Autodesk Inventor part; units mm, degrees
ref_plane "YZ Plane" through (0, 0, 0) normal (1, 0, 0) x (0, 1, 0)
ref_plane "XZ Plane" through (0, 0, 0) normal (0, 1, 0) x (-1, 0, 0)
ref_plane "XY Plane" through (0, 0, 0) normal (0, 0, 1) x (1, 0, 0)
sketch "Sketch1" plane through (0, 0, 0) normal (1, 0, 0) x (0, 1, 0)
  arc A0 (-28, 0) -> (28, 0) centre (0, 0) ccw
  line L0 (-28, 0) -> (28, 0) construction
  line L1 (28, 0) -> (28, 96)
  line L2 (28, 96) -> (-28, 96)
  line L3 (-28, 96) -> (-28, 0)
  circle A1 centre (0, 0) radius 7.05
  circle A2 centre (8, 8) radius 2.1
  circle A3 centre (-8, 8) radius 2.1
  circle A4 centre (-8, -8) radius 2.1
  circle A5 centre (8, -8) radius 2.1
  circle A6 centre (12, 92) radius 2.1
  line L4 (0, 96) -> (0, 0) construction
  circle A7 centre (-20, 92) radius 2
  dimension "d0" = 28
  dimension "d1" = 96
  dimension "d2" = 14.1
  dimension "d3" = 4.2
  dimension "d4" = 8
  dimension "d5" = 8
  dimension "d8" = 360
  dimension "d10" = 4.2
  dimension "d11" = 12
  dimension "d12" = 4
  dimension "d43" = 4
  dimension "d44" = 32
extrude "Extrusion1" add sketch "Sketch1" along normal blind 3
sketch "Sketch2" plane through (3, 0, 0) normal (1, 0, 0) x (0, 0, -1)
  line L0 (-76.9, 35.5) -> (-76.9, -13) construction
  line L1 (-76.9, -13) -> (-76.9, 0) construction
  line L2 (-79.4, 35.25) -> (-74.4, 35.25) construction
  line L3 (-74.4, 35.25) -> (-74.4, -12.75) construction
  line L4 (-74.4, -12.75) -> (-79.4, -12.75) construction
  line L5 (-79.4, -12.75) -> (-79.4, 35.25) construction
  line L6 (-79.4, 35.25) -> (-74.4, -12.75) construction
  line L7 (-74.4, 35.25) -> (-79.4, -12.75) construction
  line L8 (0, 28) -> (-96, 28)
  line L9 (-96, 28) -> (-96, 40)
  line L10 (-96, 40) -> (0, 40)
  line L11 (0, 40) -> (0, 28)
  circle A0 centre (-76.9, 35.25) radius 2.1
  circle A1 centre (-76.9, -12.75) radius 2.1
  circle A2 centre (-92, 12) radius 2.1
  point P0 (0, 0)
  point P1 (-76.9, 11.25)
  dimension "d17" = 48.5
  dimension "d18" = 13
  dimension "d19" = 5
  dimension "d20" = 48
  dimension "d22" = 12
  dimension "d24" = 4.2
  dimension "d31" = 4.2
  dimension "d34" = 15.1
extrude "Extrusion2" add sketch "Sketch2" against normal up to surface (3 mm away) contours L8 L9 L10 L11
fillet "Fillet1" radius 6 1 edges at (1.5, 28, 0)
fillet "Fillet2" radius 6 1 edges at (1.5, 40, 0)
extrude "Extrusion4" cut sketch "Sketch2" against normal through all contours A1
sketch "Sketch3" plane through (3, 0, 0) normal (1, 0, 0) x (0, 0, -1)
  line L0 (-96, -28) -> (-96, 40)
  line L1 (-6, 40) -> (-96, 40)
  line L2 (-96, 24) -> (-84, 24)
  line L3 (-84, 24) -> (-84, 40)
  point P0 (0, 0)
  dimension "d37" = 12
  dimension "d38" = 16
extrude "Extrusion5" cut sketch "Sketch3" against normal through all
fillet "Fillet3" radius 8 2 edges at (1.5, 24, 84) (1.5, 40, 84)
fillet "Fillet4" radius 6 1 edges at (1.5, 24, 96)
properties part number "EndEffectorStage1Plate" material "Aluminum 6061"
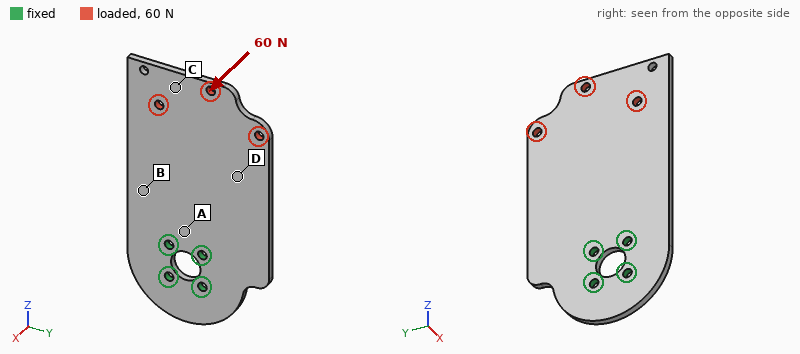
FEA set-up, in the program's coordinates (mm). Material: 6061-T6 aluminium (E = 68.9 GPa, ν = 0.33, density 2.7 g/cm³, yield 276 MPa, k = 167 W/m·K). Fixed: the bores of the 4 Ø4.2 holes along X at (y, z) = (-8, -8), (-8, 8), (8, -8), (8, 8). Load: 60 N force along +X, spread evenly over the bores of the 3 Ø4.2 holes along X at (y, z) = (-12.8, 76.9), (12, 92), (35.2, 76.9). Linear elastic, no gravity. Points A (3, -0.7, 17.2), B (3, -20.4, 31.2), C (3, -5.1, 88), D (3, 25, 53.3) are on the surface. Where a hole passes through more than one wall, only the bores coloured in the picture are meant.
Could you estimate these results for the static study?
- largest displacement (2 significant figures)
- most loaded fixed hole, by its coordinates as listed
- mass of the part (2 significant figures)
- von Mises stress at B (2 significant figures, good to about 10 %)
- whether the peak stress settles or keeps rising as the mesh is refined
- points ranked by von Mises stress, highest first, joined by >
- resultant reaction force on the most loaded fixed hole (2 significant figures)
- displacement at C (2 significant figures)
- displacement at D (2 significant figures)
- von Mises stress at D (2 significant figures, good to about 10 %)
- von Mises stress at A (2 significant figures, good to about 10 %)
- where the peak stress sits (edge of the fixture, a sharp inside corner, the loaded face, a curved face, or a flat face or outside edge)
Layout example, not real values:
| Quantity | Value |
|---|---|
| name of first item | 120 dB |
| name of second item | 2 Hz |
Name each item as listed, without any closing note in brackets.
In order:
| Quantity | Value |
|---|---|
| largest displacement | 1.0 mm |
| most loaded fixed hole, by its coordinates as listed | (8, 8) |
| mass of the part | 59 g |
| von Mises stress at B | 30 MPa |
| whether the peak stress settles or keeps rising as the mesh is refined | keeps rising |
| points ranked by von Mises stress, highest first, joined by > | A > B > D > C |
| resultant reaction force on the most loaded fixed hole | 120 N |
| displacement at C | 0.87 mm |
| displacement at D | 0.39 mm |
| von Mises stress at D | 16 MPa |
| von Mises stress at A | 41 MPa |
| where the peak stress sits | edge of the fixture |
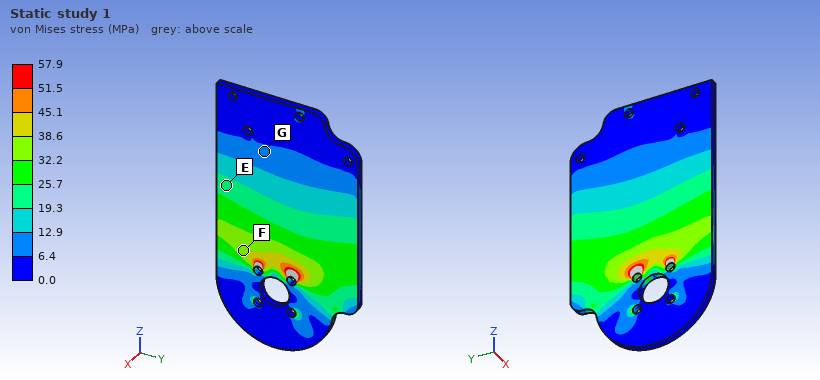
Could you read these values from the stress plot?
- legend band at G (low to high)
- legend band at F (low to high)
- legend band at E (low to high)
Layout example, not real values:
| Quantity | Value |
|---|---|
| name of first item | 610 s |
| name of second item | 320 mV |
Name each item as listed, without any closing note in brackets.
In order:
| Quantity | Value |
|---|---|
| legend band at G | 6.4 to 12.9 MPa |
| legend band at F | 32.2 to 38.6 MPa |
| legend band at E | 19.3 to 25.7 MPa |
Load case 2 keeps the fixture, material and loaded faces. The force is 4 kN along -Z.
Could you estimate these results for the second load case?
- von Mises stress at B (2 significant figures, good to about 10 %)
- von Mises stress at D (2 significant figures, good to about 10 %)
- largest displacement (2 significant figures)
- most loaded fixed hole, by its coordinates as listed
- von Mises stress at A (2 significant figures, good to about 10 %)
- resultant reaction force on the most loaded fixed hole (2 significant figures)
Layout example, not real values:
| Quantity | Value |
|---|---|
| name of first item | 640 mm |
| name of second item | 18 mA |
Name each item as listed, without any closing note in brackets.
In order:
| Quantity | Value |
|---|---|
| von Mises stress at B | 9.4 MPa |
| von Mises stress at D | 24 MPa |
| largest displacement | 74 µm |
| most loaded fixed hole, by its coordinates as listed | (8, 8) |
| von Mises stress at A | 24 MPa |
| resultant reaction force on the most loaded fixed hole | 2.5 kN |
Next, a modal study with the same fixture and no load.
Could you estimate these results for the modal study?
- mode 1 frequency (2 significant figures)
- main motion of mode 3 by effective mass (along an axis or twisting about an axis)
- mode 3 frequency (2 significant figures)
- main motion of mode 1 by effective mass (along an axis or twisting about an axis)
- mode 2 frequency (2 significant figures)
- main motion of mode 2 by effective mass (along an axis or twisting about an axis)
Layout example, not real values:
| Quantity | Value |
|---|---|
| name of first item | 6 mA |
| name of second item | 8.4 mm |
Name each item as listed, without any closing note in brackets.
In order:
| Quantity | Value |
|---|---|
| mode 1 frequency | 330 Hz |
| main motion of mode 3 by effective mass | along X |
| mode 3 frequency | 1900 Hz |
| main motion of mode 1 by effective mass | along X |
| mode 2 frequency | 890 Hz |
| main motion of mode 2 by effective mass | twisting about Z |
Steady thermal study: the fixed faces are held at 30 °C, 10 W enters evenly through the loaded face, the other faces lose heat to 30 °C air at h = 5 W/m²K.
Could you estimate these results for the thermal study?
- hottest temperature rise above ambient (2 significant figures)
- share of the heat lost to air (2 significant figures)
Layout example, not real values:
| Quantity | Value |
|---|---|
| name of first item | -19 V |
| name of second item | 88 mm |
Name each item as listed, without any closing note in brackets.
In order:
| Quantity | Value |
|---|---|
| hottest temperature rise above ambient | 25 K |
| share of the heat lost to air | 8.3 % |
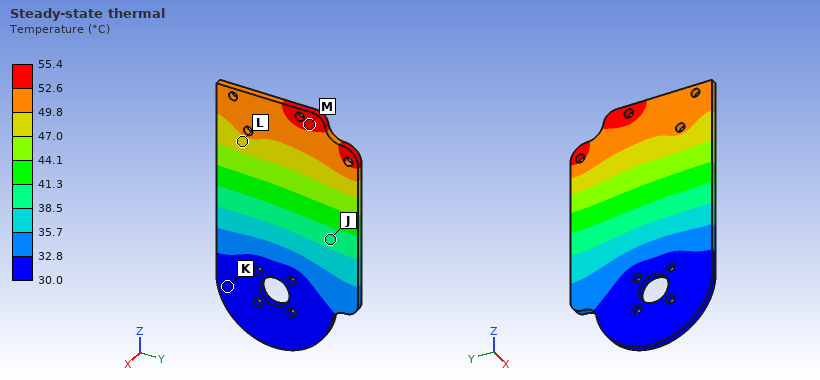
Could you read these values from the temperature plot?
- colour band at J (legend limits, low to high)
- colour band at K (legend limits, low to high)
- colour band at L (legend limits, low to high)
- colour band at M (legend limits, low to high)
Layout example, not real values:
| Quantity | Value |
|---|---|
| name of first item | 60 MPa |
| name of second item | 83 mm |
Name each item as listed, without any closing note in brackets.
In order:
| Quantity | Value |
|---|---|
| colour band at J | 38.5 to 41.3 °C |
| colour band at K | 30.0 to 32.8 °C |
| colour band at L | 47.0 to 49.8 °C |
| colour band at M | 52.6 to 55.4 °C |
